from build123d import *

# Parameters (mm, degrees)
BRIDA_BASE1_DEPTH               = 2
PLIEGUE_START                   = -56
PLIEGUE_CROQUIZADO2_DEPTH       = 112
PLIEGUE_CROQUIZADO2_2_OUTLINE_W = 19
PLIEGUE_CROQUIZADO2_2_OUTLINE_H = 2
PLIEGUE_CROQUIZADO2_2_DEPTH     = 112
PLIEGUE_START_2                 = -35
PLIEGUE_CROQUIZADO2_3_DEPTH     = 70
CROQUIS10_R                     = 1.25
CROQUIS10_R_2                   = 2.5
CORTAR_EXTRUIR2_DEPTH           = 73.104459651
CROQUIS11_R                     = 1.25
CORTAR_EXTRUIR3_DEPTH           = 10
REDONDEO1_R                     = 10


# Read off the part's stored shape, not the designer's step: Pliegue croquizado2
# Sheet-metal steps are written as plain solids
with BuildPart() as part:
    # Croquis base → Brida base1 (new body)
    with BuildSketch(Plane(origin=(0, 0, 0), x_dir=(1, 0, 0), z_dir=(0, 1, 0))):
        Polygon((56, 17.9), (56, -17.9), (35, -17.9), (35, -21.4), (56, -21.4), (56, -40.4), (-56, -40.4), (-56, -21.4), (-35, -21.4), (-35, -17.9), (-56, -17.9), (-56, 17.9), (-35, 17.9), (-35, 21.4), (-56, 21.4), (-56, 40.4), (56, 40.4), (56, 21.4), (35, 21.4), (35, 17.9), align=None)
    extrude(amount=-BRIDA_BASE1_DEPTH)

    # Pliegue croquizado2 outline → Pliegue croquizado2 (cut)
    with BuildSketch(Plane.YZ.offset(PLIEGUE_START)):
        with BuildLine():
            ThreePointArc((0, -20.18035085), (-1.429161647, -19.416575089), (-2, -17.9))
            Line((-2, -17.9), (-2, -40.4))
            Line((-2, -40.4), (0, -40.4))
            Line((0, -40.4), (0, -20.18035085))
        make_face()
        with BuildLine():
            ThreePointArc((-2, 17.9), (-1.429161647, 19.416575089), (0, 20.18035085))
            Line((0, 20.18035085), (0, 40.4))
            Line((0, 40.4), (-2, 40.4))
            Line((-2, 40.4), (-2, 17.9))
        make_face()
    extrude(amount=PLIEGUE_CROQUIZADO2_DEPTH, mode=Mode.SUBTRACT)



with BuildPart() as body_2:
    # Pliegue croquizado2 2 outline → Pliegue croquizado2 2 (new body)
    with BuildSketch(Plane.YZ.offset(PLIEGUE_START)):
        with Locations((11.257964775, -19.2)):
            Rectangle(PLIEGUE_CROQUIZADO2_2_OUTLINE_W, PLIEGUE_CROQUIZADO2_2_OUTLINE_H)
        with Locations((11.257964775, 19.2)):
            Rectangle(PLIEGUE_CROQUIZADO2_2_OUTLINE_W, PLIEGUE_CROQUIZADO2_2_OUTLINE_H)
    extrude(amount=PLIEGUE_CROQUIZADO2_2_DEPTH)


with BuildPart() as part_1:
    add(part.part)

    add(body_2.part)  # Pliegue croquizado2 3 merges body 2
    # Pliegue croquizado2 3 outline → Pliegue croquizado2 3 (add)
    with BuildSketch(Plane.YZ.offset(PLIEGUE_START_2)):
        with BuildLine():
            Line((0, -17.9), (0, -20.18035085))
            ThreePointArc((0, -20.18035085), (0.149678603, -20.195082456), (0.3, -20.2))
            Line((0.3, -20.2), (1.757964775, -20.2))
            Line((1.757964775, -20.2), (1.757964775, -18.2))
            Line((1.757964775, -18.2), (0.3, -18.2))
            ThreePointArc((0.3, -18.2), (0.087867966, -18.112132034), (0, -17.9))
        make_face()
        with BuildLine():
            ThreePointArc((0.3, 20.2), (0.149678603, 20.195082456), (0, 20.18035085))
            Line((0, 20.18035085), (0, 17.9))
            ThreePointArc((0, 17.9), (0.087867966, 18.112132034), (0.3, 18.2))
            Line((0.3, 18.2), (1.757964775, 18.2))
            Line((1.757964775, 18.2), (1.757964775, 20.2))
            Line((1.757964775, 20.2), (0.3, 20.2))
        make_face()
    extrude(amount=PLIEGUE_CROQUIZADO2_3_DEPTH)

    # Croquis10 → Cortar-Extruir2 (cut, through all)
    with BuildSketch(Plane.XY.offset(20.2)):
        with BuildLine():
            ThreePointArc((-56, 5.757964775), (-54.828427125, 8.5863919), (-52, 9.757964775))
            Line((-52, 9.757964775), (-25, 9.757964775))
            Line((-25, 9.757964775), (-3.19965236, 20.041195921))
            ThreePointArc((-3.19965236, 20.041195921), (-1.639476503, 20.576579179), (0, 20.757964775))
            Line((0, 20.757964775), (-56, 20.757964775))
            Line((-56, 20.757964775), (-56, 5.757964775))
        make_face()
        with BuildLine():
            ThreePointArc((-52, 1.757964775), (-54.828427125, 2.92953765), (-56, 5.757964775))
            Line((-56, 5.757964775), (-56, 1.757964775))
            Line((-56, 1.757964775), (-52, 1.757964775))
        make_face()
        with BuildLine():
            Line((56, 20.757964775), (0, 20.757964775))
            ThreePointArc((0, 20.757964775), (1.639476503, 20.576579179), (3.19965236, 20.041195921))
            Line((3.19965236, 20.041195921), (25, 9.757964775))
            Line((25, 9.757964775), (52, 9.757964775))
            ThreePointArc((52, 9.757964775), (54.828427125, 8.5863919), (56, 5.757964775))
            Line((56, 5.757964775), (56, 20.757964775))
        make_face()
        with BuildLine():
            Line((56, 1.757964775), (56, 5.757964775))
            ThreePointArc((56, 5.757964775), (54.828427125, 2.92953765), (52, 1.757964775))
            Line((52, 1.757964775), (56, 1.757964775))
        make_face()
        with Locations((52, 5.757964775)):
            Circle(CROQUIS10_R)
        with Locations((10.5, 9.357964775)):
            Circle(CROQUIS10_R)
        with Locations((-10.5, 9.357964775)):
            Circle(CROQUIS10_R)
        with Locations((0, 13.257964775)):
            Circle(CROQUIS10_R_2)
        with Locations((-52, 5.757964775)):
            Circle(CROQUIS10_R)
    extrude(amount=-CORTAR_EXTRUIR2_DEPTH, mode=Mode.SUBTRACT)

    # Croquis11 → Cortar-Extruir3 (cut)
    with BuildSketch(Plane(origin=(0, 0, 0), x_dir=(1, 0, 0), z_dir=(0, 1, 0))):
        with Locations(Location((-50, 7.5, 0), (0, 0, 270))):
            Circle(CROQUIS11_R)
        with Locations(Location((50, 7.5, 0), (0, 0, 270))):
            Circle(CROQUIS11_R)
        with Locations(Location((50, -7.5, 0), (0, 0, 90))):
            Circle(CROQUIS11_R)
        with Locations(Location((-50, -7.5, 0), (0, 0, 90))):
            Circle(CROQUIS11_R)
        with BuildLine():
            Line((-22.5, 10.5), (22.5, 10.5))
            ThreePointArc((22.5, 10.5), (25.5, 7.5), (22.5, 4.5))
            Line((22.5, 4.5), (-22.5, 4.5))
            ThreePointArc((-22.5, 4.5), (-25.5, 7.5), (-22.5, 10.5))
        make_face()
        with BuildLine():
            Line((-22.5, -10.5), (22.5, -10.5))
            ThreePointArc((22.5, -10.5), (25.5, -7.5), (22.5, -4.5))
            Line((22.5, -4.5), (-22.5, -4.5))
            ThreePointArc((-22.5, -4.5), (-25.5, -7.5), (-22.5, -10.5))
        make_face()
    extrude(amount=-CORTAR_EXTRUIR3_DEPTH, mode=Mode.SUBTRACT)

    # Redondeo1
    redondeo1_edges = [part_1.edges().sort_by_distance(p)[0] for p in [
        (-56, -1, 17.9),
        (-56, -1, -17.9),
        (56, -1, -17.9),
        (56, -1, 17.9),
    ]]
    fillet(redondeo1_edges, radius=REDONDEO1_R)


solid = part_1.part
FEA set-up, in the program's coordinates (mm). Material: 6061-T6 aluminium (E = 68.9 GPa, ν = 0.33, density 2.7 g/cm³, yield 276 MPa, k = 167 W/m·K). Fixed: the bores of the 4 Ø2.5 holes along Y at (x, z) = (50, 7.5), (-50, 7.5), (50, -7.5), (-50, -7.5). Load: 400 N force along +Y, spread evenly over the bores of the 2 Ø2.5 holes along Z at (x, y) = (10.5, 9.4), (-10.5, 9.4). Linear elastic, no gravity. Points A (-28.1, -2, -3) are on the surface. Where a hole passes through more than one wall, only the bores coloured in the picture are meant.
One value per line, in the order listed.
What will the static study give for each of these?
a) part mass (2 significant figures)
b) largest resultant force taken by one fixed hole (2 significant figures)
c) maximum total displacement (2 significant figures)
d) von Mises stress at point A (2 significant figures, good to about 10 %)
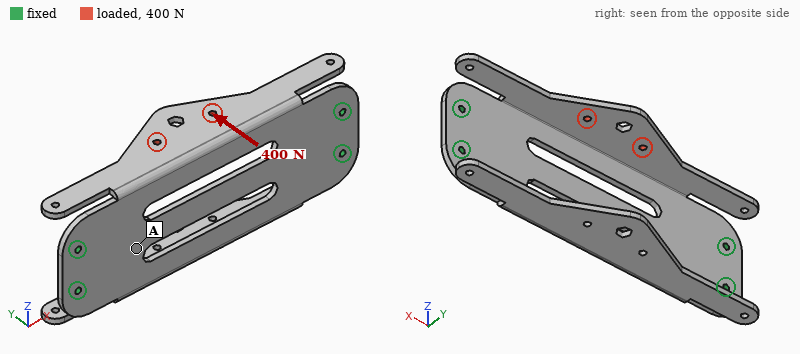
33 g
370 N
0.71 mm
37 MPa
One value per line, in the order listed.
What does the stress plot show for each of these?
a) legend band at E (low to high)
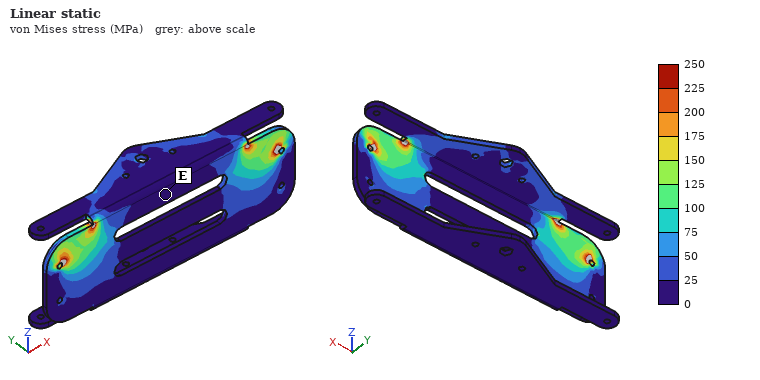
0 to 25 MPa
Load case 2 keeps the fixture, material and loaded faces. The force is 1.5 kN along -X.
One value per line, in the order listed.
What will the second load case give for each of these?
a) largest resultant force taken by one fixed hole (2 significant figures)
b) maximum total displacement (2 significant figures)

830 N
0.55 mm
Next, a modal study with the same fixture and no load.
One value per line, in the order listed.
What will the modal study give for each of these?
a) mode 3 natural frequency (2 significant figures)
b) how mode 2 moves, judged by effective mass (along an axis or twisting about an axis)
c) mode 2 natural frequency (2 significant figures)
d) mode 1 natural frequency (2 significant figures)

1700 Hz
along Y
1500 Hz
1300 Hz
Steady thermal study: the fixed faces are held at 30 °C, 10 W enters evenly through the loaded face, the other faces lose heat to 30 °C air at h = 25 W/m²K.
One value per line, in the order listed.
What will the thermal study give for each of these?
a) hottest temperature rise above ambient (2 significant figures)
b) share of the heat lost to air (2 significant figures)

31 K
29 %
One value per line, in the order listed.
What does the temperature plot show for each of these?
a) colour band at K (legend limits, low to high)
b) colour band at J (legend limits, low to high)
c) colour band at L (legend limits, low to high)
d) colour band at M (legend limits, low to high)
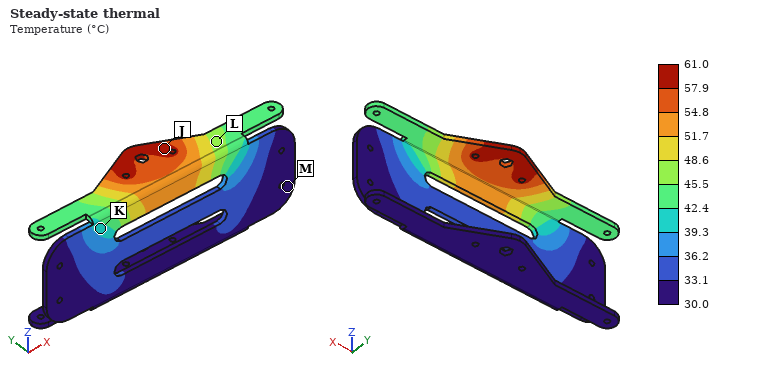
39.3 to 42.4 °C
57.9 to 61.0 °C
45.5 to 48.6 °C
30.0 to 33.1 °C
